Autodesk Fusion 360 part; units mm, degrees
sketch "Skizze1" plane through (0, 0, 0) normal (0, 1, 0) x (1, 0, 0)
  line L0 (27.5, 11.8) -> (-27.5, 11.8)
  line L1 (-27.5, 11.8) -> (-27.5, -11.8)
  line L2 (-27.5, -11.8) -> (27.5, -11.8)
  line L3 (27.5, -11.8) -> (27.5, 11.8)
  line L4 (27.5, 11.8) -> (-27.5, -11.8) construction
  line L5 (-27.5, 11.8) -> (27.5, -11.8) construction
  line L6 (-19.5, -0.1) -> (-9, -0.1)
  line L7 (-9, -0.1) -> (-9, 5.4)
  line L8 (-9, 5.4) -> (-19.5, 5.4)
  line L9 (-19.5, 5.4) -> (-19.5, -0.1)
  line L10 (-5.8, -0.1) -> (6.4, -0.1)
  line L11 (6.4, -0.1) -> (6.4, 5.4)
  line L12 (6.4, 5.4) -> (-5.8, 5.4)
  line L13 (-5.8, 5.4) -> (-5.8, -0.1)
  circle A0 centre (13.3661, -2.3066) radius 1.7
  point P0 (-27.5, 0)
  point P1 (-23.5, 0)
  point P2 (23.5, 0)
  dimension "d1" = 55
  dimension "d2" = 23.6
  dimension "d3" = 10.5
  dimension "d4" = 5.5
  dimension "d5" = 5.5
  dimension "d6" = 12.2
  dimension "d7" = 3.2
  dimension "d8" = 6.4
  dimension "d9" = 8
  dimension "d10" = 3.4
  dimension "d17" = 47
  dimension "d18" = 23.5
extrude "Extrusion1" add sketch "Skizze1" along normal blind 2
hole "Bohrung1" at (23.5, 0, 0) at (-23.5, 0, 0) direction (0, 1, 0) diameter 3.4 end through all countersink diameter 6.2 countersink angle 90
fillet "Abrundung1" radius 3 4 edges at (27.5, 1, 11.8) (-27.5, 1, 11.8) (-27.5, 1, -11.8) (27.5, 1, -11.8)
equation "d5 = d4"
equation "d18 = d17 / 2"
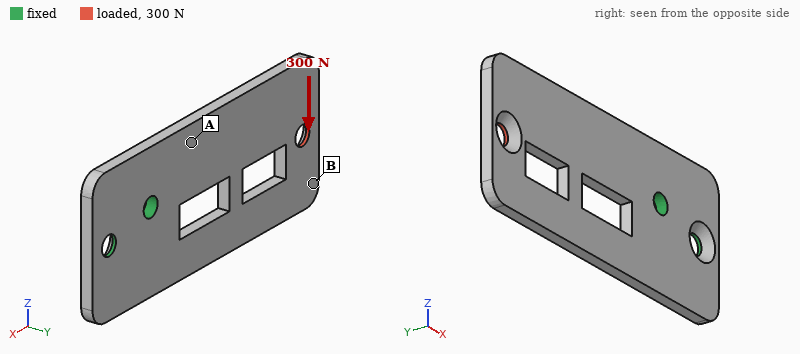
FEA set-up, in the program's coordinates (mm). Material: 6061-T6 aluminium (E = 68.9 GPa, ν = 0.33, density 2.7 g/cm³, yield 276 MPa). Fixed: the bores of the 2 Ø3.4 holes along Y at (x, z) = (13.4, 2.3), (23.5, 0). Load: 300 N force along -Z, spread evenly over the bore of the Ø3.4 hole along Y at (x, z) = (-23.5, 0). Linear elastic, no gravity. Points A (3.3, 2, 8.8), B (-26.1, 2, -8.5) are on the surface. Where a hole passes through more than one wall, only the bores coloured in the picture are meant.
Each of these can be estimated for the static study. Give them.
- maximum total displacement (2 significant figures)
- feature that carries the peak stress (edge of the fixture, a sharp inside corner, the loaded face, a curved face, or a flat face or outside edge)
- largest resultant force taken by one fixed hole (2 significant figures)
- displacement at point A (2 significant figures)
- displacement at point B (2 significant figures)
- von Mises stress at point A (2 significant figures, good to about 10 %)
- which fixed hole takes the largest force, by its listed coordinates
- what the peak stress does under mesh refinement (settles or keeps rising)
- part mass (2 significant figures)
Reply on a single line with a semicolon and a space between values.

0.16 mm; edge of the fixture; 1.0 kN; 0.032 mm; 0.15 mm; 47 MPa; (13.4, 2.3); keeps rising; 6.1 g
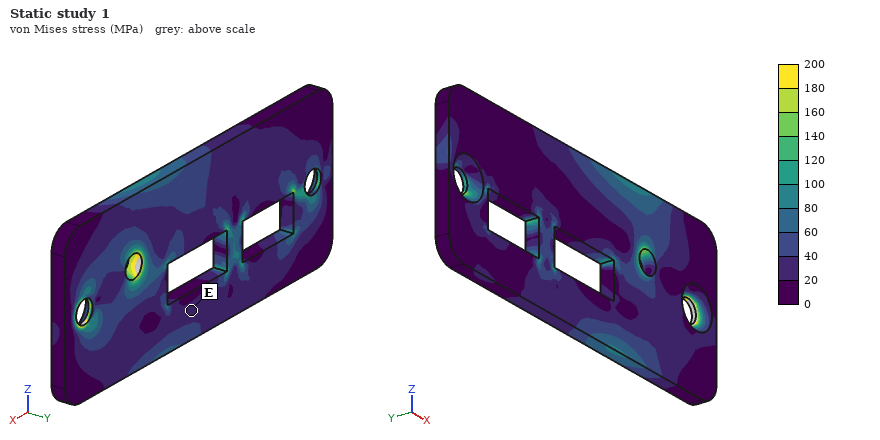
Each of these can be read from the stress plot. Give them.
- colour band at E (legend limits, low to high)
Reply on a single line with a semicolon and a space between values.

20 to 40 MPa
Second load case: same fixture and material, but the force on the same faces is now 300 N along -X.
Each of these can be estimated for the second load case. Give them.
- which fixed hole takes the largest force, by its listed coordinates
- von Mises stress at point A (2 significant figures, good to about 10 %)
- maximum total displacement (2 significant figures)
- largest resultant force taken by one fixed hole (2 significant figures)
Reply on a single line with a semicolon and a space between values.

(13.4, 2.3); 23 MPa; 0.20 mm; 230 N
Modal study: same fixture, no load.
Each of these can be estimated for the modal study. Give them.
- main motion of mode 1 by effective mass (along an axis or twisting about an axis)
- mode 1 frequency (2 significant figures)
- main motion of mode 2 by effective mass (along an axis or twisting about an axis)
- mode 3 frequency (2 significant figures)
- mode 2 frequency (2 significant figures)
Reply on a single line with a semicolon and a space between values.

along Y; 970 Hz; twisting about X; 5700 Hz; 2900 Hz
